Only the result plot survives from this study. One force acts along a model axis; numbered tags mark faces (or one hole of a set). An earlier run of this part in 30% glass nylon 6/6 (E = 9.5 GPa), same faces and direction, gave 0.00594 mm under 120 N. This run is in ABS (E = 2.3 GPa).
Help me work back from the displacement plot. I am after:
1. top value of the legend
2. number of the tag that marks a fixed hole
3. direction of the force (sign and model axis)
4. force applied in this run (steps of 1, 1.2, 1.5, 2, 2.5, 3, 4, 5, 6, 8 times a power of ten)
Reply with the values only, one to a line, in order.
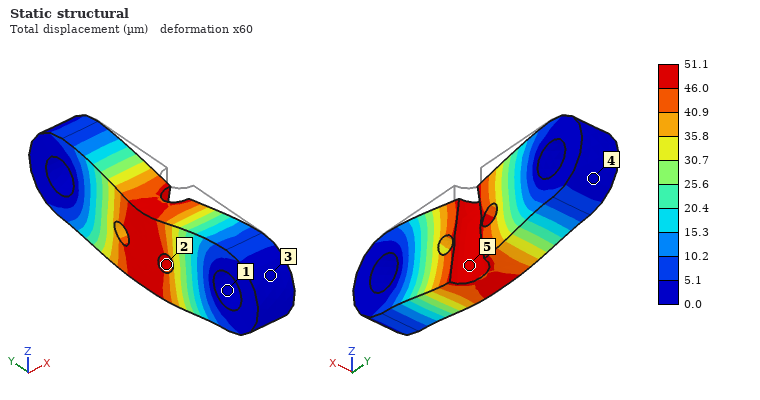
51.1 µm
1
-Z
250 N
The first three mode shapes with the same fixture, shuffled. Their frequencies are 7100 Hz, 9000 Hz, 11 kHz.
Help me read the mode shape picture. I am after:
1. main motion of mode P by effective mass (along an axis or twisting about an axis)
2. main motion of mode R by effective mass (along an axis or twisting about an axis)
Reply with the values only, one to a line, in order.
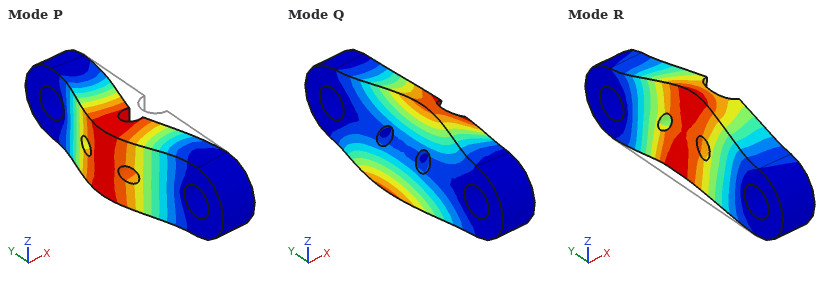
along X
along Z
